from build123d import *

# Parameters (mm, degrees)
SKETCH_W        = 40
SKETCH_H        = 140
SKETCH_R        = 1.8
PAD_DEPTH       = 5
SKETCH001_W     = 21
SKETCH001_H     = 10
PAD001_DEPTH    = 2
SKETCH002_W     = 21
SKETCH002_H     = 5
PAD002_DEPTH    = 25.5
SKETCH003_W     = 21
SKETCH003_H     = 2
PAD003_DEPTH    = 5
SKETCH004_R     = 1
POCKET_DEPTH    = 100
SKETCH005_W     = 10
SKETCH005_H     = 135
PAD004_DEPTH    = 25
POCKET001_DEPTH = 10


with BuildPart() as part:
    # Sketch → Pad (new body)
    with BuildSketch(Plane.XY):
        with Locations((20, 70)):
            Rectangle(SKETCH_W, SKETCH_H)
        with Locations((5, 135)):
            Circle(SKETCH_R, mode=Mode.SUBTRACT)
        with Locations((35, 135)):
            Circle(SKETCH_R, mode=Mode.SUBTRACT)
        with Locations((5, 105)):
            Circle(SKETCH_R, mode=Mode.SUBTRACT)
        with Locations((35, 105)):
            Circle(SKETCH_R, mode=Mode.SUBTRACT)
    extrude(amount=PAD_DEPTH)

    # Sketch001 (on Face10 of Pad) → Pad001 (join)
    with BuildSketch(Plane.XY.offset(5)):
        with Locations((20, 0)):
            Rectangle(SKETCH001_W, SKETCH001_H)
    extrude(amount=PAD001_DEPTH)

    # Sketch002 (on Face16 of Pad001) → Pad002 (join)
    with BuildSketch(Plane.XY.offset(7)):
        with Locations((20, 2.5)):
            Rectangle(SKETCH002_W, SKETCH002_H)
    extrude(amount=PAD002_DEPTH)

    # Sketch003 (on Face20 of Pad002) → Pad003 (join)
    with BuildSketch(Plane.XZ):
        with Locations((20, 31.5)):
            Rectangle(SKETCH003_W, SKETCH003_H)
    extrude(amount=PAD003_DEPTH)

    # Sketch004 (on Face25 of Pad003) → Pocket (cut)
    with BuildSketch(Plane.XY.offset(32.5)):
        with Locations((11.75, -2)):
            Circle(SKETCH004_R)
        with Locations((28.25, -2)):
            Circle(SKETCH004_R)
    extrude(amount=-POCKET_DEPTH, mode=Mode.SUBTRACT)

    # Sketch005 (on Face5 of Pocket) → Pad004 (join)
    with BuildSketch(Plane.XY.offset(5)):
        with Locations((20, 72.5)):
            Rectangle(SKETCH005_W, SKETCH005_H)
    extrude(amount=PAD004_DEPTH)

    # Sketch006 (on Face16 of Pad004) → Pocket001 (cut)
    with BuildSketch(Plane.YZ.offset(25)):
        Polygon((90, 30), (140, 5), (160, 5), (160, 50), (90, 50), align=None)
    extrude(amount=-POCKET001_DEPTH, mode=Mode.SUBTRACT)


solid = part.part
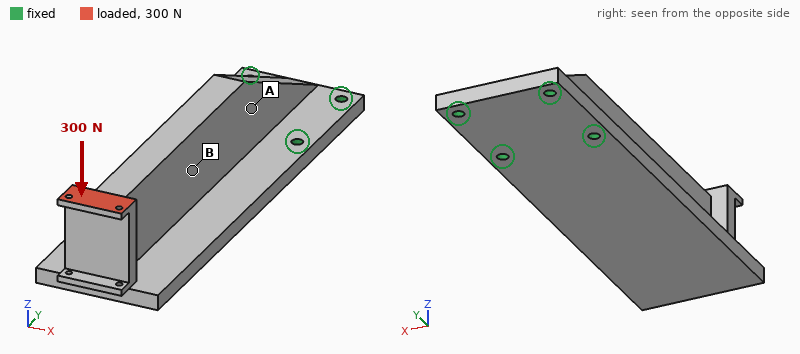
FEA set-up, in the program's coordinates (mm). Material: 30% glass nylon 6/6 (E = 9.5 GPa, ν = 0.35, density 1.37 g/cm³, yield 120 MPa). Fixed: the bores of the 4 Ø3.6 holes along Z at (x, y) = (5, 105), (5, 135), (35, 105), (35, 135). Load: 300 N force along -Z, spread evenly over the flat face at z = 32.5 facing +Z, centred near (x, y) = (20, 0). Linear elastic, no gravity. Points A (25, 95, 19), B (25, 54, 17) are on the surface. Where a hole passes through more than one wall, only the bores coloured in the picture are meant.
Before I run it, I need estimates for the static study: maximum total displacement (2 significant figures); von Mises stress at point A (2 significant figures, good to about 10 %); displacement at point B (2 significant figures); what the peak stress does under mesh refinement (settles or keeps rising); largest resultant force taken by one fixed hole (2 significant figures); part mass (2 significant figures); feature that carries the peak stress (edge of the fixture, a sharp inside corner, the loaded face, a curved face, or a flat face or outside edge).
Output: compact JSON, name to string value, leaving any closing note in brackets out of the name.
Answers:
{"maximum total displacement": "1.6 mm", "von Mises stress at point A": "11 MPa", "displacement at point B": "0.69 mm", "what the peak stress does under mesh refinement": "keeps rising", "largest resultant force taken by one fixed hole": "730 N", "part mass": "80 g", "feature that carries the peak stress": "edge of the fixture"}
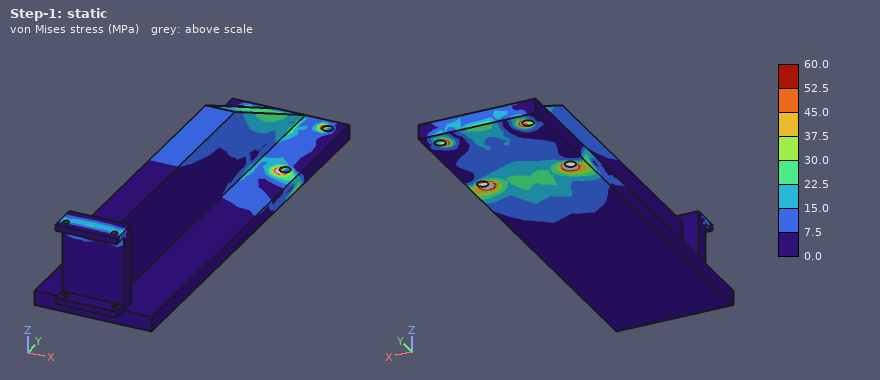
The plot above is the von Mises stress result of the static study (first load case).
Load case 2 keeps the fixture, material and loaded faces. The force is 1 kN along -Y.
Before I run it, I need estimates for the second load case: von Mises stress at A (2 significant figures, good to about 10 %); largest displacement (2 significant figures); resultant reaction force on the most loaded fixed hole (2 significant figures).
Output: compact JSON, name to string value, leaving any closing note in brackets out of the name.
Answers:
{"von Mises stress at A": "12 MPa", "largest displacement": "1.6 mm", "resultant reaction force on the most loaded fixed hole": "610 N"}
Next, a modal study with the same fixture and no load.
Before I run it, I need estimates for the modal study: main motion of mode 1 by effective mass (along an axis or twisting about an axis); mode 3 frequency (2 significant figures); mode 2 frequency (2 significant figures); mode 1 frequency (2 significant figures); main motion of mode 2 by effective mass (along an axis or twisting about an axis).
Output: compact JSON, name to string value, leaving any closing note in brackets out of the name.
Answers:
{"main motion of mode 1 by effective mass": "along Z", "mode 3 frequency": "1400 Hz", "mode 2 frequency": "790 Hz", "mode 1 frequency": "460 Hz", "main motion of mode 2 by effective mass": "along X"}
